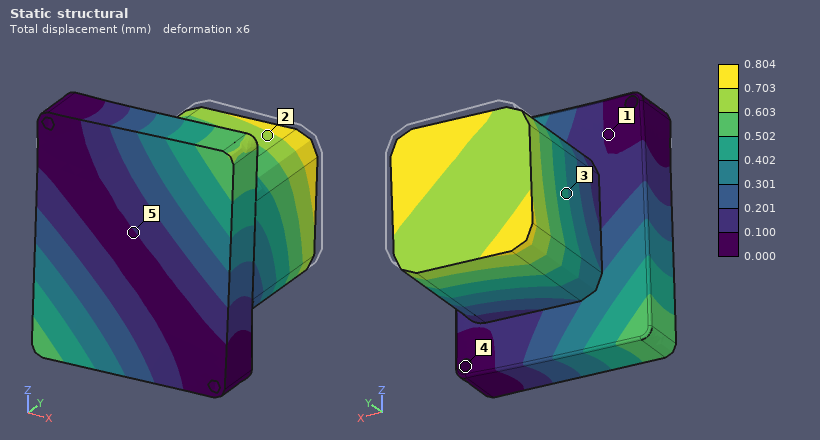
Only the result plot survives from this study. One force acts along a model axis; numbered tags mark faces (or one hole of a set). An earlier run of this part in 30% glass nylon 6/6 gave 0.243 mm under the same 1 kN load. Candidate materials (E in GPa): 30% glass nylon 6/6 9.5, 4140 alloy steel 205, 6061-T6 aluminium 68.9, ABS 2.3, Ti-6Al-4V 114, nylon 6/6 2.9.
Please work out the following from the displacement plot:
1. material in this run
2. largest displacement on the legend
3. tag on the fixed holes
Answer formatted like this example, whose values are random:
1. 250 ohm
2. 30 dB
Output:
1. nylon 6/6
2. 0.804 mm
3. 4
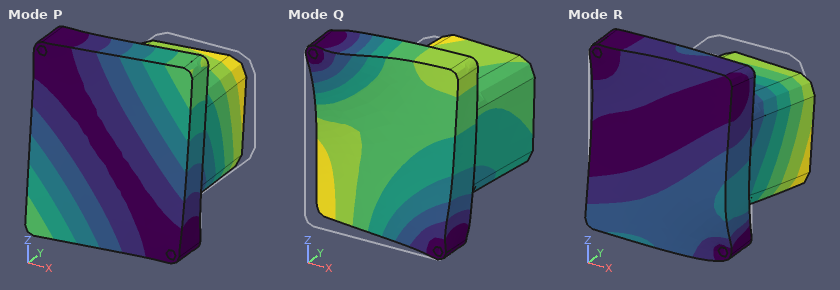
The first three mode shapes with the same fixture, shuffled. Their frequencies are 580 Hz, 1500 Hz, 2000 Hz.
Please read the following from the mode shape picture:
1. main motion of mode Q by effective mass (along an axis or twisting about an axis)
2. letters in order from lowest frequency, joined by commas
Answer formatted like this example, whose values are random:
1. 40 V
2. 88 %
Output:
1. along Y
2. P, Q, R
